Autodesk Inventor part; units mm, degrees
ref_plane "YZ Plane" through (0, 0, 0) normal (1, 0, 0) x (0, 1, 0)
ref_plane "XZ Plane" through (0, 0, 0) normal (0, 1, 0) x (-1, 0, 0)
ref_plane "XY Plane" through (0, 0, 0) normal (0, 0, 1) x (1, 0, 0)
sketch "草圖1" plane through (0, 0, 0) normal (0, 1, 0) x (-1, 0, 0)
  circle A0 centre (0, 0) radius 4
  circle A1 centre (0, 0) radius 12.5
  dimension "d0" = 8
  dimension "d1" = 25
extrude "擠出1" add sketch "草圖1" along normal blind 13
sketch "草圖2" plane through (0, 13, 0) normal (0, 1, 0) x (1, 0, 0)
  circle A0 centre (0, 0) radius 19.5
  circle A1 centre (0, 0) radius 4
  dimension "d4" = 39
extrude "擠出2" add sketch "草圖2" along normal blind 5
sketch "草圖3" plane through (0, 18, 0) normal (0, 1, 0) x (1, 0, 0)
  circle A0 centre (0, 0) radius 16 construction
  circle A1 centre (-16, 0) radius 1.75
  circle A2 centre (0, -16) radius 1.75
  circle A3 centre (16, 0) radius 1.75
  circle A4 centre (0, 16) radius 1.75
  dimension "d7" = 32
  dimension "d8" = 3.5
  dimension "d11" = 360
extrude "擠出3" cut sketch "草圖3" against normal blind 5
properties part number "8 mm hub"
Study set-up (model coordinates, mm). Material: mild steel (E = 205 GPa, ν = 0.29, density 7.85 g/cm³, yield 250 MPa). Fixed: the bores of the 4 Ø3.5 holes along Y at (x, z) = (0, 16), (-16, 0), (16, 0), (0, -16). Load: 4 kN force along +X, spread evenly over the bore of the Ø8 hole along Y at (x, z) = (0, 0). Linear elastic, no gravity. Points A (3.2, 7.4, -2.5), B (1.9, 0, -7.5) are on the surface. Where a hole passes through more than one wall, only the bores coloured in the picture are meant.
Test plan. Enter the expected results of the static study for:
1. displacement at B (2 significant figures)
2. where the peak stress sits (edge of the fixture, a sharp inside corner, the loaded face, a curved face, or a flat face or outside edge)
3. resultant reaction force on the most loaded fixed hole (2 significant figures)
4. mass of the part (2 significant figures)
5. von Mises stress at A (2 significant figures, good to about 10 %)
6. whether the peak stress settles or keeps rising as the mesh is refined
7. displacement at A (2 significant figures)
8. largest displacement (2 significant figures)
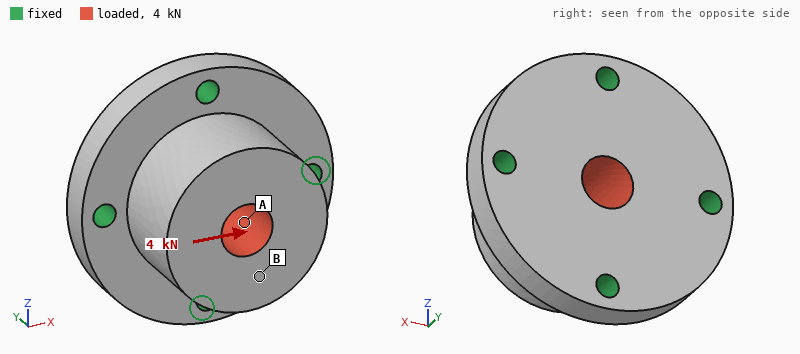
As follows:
3.0 µm
edge of the fixture
1.5 kN
88 g
15 MPa
keeps rising
2.2 µm
3.5 µm
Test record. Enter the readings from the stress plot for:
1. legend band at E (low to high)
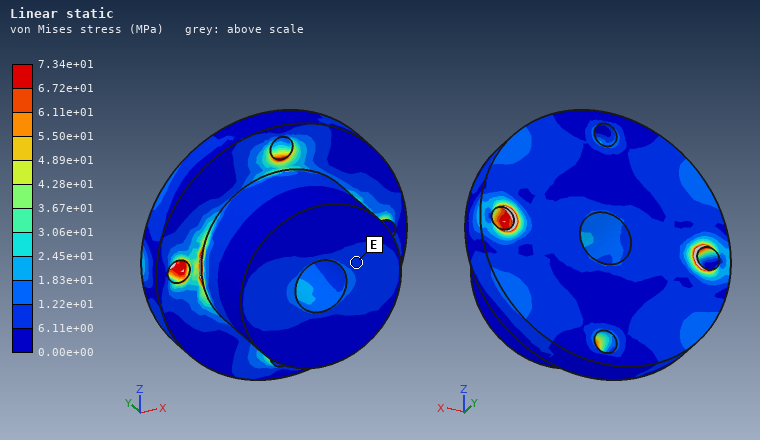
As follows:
6.11e+00 to 1.22e+01 MPa
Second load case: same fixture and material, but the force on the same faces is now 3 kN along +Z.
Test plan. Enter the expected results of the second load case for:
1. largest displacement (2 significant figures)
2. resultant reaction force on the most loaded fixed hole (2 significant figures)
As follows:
2.6 µm
1.2 kN
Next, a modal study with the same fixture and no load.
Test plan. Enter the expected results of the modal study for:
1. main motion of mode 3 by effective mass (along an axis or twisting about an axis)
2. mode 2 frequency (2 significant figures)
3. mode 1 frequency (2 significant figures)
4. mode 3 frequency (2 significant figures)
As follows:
along Y
24 kHz
24 kHz
27 kHz
